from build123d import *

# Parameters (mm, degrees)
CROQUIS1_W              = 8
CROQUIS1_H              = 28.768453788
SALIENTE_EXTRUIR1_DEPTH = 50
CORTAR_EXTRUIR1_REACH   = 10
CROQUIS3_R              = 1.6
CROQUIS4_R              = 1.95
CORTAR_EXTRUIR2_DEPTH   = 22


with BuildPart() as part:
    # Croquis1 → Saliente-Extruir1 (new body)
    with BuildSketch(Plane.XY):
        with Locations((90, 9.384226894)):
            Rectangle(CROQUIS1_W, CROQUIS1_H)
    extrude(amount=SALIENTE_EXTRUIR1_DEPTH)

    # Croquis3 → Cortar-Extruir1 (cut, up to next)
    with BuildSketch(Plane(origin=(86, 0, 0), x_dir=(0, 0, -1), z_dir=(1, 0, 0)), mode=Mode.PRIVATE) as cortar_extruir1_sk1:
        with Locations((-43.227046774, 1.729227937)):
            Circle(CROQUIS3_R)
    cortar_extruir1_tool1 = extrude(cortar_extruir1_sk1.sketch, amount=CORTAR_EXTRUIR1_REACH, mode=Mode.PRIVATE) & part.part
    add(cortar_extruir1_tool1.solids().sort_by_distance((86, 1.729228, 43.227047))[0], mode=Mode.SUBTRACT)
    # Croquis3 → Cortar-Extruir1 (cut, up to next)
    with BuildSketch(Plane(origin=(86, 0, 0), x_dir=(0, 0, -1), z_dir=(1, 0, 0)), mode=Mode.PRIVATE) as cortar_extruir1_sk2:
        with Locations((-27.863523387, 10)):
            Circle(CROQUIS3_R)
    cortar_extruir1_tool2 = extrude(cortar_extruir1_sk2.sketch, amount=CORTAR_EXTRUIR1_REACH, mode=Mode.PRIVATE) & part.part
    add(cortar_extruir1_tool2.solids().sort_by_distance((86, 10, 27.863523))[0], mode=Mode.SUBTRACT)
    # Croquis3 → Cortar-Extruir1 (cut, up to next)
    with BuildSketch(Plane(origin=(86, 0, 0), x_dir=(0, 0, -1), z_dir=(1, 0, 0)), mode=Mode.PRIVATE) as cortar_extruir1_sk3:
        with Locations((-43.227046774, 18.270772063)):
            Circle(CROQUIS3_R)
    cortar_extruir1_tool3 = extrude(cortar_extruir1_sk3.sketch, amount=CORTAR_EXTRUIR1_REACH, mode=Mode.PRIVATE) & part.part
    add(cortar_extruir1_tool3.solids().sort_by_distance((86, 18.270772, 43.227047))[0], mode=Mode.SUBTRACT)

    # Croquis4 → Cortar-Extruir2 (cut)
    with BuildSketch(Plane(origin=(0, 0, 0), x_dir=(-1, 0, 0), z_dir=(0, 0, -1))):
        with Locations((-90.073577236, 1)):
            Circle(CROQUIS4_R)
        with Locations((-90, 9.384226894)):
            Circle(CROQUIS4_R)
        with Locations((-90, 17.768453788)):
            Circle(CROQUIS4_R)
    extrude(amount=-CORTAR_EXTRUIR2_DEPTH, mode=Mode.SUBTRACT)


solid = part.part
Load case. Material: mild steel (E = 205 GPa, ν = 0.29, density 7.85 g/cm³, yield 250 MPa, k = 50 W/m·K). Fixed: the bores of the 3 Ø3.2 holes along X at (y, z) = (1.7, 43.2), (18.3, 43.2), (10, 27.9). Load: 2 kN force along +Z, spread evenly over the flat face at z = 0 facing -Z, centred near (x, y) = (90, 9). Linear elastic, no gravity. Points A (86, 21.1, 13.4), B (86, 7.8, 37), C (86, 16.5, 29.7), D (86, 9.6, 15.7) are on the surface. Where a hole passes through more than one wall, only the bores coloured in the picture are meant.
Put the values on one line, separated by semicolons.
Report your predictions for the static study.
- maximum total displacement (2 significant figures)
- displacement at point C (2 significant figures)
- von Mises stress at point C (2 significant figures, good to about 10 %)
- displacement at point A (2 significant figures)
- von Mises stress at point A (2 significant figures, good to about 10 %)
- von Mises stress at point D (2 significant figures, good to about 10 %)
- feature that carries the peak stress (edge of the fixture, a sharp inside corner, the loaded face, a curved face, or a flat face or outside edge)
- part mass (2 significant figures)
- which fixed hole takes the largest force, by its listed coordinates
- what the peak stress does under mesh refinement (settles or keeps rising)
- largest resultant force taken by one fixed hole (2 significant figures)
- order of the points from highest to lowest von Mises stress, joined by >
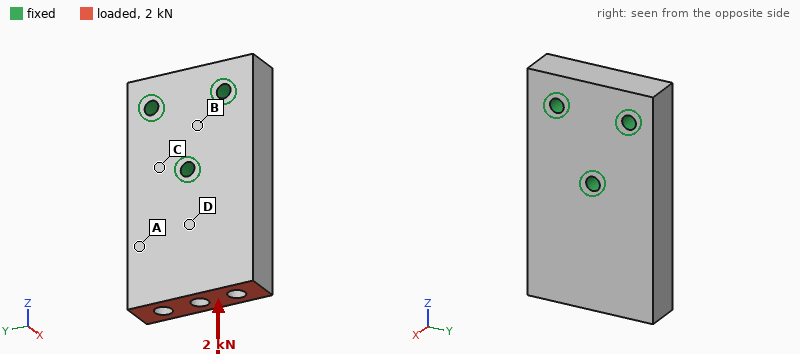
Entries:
1.8 µm; 0.27 µm; 5.9 MPa; 0.99 µm; 9.5 MPa; 13 MPa; edge of the fixture; 83 g; (10, 27.9); keeps rising; 1.2 kN; D > A > C > B
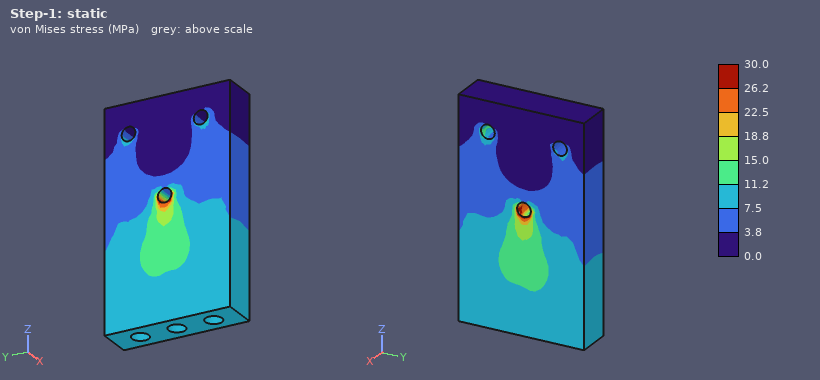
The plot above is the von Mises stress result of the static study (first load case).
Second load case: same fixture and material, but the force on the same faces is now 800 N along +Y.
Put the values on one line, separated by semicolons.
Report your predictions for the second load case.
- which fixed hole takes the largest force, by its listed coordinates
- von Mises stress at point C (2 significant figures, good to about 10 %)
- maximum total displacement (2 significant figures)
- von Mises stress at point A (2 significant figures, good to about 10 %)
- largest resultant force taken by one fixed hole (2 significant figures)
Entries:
(10, 27.9); 11 MPa; 7.4 µm; 9.9 MPa; 1.3 kN
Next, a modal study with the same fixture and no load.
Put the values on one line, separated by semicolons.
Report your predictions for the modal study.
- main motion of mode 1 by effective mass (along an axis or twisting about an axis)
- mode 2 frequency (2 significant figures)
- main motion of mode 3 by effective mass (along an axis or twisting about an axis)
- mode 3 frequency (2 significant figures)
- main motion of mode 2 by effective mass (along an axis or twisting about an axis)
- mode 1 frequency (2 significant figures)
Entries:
along X; 13 kHz; along Y; 14 kHz; twisting about Z; 7400 Hz
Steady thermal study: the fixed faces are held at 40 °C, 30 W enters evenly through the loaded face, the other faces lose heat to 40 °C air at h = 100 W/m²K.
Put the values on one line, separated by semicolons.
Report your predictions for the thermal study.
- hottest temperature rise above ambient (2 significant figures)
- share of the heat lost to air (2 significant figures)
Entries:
71 K; 37 %
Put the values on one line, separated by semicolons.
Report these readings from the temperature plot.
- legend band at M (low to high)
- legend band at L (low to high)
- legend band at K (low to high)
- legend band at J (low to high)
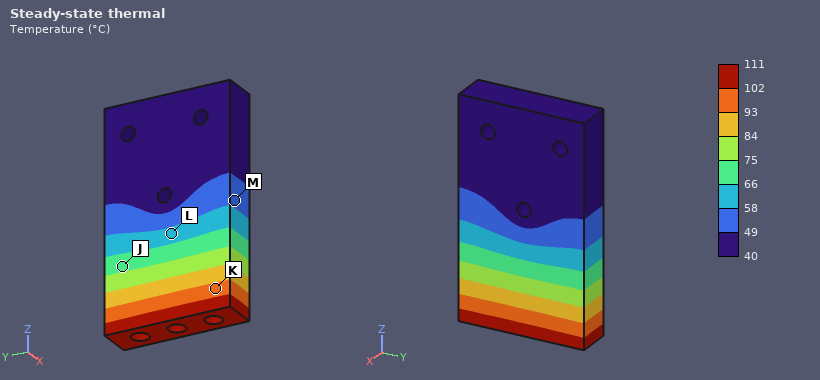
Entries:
49 to 58 °C; 58 to 66 °C; 93 to 102 °C; 66 to 75 °C
